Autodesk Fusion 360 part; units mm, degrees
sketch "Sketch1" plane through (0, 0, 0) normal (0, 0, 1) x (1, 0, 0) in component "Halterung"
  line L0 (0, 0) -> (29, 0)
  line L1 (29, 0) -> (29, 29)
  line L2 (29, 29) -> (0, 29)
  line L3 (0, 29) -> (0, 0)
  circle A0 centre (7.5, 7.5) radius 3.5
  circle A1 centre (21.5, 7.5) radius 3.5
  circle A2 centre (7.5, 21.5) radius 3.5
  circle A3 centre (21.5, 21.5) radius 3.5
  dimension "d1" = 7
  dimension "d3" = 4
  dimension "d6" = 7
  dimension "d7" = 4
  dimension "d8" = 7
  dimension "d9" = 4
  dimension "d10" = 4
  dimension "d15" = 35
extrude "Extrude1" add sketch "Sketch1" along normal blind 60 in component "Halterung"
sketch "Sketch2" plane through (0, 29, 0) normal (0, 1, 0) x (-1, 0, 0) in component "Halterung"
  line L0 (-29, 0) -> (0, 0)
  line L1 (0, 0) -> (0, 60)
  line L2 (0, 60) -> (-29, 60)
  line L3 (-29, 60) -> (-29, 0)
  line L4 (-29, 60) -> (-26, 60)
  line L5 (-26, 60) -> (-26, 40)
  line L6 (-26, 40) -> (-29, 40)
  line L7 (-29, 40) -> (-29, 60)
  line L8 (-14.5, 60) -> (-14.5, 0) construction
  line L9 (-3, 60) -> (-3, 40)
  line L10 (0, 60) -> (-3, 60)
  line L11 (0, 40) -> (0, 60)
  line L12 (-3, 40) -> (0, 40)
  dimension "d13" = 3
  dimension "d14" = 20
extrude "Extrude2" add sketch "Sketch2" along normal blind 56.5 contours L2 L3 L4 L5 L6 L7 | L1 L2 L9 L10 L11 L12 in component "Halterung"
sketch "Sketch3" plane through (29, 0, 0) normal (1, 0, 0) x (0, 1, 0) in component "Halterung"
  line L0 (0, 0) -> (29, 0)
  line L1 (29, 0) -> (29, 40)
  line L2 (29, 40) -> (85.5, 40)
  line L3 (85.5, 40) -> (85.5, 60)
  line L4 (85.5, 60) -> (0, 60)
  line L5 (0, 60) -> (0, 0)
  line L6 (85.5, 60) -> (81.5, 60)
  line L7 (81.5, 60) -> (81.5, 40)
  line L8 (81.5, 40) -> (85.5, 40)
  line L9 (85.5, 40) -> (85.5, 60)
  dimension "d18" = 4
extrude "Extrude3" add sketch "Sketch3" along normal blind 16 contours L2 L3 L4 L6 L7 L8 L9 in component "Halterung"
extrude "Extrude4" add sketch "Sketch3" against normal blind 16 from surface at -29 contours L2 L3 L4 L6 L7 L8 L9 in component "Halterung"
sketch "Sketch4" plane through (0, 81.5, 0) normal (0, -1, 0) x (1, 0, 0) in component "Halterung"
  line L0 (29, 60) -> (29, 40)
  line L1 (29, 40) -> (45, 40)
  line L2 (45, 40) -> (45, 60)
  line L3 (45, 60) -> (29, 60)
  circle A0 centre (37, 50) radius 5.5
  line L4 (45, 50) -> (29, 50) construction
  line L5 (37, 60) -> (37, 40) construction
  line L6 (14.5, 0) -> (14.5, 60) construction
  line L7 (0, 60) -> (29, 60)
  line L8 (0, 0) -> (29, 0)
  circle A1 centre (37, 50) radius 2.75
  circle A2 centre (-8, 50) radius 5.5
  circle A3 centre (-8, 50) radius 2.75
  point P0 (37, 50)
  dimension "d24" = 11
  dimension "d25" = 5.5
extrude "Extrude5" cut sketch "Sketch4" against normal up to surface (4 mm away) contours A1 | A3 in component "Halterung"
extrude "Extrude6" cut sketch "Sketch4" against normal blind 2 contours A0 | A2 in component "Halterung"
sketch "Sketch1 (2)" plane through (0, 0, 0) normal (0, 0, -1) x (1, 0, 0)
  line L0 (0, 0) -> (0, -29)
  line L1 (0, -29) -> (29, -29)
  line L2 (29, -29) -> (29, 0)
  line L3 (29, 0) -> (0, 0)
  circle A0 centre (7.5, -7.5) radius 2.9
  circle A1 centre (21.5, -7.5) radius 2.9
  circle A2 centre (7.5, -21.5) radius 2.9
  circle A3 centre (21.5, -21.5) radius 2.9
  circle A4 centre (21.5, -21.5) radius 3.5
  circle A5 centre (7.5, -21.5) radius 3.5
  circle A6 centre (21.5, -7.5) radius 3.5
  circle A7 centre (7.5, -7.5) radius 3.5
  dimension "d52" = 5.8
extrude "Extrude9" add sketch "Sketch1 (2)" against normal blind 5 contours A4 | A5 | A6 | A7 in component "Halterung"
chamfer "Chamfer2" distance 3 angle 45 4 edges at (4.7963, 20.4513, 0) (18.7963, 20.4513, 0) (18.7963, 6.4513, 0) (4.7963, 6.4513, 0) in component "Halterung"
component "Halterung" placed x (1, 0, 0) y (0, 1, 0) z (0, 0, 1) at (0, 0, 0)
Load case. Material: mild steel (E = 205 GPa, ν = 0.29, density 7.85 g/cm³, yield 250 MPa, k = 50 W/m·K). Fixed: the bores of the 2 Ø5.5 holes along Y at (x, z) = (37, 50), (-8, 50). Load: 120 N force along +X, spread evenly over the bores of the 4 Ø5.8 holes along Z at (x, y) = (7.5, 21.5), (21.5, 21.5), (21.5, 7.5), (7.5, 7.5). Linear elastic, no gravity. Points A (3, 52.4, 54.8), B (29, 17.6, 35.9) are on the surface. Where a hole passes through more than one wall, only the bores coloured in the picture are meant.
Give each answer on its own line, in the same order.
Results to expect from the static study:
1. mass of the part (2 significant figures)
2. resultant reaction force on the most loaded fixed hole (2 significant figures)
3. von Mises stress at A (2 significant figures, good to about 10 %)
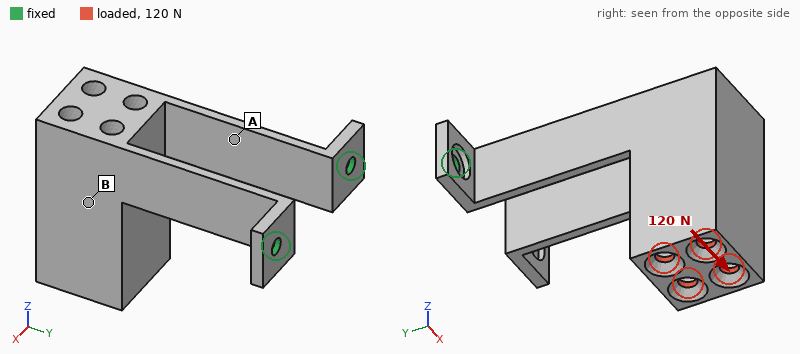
390 g
260 N
11 MPa
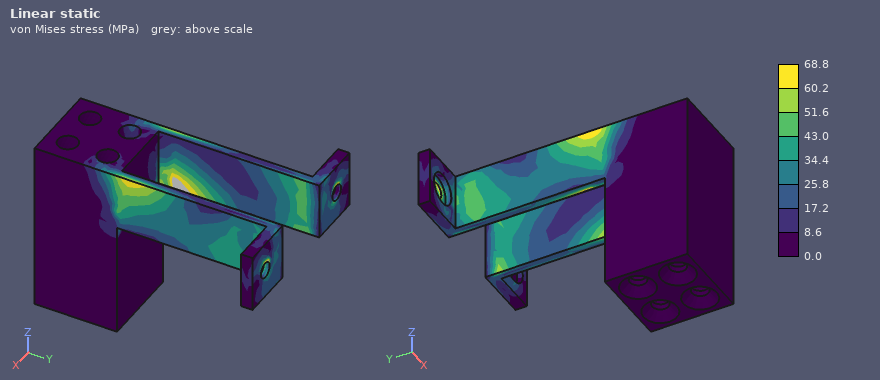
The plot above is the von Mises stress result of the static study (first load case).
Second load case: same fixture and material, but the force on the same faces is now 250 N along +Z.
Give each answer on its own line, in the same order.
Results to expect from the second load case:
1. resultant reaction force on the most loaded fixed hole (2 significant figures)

130 N
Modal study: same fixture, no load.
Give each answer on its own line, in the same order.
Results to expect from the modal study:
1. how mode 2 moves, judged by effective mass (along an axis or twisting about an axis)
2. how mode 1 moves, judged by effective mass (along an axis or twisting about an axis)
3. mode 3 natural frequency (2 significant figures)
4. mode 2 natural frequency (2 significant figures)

along X
along Z
760 Hz
270 Hz
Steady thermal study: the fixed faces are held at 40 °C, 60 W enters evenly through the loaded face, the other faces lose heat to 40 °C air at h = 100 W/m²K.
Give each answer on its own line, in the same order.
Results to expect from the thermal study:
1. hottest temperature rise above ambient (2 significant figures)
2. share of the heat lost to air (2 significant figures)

76 K
98 %
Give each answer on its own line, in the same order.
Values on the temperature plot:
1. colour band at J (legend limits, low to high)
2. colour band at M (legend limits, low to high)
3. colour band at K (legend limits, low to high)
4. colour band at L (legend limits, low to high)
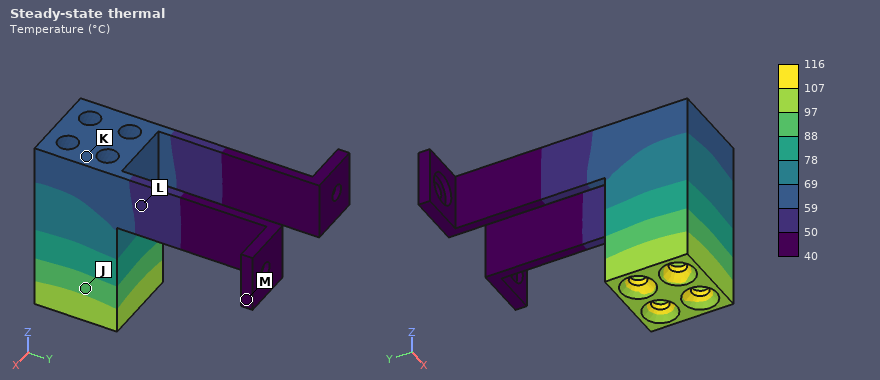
88 to 97 °C
40 to 50 °C
59 to 69 °C
50 to 59 °C
